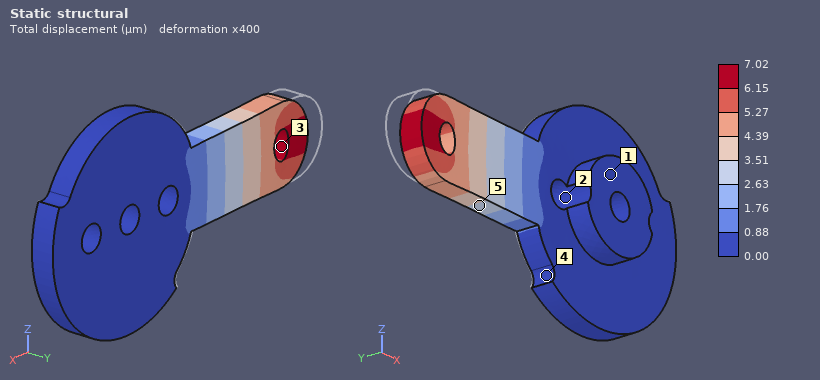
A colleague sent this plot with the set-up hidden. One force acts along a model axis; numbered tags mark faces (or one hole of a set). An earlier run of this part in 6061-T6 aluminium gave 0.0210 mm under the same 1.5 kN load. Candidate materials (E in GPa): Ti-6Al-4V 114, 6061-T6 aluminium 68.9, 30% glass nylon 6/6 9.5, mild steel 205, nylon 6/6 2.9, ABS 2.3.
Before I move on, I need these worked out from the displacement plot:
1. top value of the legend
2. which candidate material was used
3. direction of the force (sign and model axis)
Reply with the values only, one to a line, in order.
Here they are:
7.02 µm
mild steel
+X
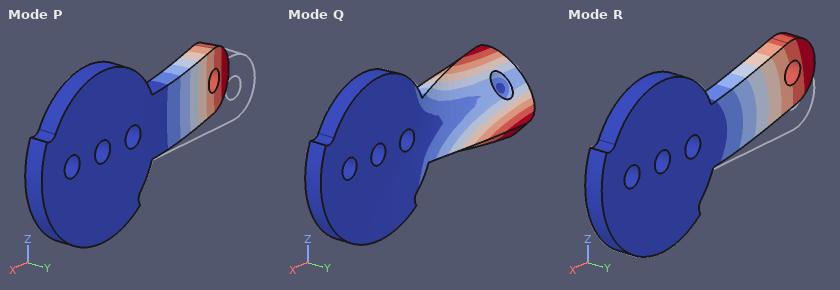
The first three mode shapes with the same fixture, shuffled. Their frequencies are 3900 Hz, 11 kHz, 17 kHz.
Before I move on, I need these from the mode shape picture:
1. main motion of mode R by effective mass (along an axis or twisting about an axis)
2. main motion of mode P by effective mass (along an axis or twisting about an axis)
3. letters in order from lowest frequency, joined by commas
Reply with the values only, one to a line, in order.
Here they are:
along Z
along Y
P, R, Q
